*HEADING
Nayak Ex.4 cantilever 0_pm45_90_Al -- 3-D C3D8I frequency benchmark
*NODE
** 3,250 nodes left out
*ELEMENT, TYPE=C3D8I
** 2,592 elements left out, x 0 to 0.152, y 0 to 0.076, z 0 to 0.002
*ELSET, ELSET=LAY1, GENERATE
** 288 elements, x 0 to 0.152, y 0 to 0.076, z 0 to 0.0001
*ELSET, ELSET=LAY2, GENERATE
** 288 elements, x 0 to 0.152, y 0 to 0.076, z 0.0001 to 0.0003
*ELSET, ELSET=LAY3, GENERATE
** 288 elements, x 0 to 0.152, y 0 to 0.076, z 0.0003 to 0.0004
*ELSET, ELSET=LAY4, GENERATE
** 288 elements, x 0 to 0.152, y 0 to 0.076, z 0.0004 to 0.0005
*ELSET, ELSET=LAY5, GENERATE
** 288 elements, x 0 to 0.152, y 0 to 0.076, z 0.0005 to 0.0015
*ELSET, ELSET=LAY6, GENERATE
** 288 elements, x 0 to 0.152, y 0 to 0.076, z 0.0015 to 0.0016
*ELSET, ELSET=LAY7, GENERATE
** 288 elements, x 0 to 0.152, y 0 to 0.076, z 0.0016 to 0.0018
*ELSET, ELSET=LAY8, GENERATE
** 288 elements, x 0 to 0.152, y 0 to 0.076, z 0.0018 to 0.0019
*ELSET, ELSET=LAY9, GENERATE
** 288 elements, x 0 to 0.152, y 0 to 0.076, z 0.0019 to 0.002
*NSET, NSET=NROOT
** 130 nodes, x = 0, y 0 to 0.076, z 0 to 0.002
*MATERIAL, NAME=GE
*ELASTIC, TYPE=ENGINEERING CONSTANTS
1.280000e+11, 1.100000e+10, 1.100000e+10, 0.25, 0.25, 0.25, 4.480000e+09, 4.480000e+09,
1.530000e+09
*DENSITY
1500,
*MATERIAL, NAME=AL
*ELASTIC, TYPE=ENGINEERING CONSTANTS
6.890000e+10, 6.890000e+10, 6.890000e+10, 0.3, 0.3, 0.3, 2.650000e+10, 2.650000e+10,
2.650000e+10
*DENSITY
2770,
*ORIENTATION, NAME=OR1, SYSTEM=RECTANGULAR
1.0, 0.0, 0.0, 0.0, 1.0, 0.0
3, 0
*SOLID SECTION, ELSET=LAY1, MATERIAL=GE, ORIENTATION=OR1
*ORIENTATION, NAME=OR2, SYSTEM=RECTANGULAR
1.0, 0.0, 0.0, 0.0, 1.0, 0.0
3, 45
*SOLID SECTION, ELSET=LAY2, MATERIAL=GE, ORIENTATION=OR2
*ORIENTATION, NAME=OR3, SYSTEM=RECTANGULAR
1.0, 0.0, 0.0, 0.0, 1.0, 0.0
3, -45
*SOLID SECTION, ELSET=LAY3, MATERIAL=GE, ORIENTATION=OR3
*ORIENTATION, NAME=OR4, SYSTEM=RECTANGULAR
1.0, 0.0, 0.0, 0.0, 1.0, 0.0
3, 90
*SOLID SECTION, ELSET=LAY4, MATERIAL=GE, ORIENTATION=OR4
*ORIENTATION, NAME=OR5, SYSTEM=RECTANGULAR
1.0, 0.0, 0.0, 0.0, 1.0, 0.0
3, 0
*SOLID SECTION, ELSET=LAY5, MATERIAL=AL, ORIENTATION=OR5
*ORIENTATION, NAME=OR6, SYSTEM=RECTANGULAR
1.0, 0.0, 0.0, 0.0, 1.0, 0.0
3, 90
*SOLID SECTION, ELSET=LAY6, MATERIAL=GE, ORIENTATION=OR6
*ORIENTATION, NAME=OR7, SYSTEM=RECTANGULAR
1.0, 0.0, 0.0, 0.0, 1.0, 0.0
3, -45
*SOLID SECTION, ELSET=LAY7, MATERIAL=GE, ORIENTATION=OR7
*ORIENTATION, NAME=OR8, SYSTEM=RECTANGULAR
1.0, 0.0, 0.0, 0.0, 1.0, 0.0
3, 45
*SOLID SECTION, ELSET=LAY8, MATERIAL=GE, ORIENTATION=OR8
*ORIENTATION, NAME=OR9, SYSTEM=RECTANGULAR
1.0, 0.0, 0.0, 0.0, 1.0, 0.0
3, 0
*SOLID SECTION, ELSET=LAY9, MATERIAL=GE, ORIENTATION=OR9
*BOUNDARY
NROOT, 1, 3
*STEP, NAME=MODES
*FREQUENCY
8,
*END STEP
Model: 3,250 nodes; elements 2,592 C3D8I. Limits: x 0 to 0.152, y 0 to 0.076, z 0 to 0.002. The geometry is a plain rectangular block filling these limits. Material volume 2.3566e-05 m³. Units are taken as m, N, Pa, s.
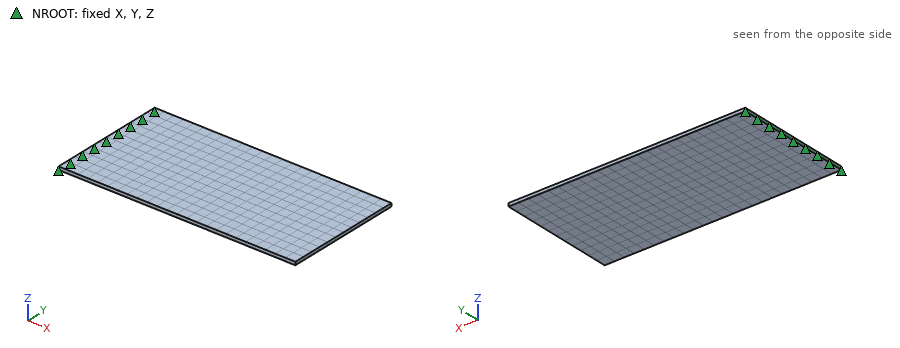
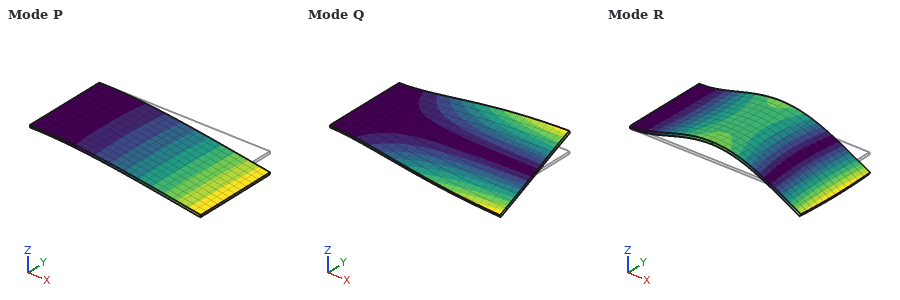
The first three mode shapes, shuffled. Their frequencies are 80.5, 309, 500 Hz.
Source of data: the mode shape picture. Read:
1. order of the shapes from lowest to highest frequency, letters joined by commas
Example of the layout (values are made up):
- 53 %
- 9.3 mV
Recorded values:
- P, Q, R
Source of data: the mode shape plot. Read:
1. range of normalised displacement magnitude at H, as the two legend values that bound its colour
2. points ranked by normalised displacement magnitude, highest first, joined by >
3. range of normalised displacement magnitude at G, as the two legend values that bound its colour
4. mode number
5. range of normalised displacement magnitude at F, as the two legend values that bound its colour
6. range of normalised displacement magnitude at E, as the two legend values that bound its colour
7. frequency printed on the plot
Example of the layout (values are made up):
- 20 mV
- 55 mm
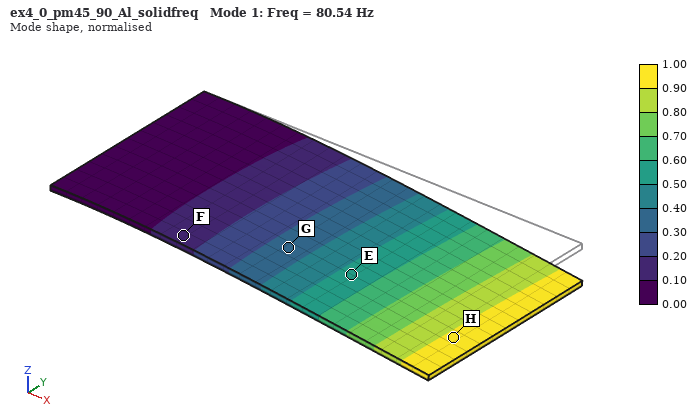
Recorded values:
- 0.90 to 1.00
- H > E > G > F
- 0.30 to 0.40
- 1
- 0.10 to 0.20
- 0.50 to 0.60
- 80.54 Hz
